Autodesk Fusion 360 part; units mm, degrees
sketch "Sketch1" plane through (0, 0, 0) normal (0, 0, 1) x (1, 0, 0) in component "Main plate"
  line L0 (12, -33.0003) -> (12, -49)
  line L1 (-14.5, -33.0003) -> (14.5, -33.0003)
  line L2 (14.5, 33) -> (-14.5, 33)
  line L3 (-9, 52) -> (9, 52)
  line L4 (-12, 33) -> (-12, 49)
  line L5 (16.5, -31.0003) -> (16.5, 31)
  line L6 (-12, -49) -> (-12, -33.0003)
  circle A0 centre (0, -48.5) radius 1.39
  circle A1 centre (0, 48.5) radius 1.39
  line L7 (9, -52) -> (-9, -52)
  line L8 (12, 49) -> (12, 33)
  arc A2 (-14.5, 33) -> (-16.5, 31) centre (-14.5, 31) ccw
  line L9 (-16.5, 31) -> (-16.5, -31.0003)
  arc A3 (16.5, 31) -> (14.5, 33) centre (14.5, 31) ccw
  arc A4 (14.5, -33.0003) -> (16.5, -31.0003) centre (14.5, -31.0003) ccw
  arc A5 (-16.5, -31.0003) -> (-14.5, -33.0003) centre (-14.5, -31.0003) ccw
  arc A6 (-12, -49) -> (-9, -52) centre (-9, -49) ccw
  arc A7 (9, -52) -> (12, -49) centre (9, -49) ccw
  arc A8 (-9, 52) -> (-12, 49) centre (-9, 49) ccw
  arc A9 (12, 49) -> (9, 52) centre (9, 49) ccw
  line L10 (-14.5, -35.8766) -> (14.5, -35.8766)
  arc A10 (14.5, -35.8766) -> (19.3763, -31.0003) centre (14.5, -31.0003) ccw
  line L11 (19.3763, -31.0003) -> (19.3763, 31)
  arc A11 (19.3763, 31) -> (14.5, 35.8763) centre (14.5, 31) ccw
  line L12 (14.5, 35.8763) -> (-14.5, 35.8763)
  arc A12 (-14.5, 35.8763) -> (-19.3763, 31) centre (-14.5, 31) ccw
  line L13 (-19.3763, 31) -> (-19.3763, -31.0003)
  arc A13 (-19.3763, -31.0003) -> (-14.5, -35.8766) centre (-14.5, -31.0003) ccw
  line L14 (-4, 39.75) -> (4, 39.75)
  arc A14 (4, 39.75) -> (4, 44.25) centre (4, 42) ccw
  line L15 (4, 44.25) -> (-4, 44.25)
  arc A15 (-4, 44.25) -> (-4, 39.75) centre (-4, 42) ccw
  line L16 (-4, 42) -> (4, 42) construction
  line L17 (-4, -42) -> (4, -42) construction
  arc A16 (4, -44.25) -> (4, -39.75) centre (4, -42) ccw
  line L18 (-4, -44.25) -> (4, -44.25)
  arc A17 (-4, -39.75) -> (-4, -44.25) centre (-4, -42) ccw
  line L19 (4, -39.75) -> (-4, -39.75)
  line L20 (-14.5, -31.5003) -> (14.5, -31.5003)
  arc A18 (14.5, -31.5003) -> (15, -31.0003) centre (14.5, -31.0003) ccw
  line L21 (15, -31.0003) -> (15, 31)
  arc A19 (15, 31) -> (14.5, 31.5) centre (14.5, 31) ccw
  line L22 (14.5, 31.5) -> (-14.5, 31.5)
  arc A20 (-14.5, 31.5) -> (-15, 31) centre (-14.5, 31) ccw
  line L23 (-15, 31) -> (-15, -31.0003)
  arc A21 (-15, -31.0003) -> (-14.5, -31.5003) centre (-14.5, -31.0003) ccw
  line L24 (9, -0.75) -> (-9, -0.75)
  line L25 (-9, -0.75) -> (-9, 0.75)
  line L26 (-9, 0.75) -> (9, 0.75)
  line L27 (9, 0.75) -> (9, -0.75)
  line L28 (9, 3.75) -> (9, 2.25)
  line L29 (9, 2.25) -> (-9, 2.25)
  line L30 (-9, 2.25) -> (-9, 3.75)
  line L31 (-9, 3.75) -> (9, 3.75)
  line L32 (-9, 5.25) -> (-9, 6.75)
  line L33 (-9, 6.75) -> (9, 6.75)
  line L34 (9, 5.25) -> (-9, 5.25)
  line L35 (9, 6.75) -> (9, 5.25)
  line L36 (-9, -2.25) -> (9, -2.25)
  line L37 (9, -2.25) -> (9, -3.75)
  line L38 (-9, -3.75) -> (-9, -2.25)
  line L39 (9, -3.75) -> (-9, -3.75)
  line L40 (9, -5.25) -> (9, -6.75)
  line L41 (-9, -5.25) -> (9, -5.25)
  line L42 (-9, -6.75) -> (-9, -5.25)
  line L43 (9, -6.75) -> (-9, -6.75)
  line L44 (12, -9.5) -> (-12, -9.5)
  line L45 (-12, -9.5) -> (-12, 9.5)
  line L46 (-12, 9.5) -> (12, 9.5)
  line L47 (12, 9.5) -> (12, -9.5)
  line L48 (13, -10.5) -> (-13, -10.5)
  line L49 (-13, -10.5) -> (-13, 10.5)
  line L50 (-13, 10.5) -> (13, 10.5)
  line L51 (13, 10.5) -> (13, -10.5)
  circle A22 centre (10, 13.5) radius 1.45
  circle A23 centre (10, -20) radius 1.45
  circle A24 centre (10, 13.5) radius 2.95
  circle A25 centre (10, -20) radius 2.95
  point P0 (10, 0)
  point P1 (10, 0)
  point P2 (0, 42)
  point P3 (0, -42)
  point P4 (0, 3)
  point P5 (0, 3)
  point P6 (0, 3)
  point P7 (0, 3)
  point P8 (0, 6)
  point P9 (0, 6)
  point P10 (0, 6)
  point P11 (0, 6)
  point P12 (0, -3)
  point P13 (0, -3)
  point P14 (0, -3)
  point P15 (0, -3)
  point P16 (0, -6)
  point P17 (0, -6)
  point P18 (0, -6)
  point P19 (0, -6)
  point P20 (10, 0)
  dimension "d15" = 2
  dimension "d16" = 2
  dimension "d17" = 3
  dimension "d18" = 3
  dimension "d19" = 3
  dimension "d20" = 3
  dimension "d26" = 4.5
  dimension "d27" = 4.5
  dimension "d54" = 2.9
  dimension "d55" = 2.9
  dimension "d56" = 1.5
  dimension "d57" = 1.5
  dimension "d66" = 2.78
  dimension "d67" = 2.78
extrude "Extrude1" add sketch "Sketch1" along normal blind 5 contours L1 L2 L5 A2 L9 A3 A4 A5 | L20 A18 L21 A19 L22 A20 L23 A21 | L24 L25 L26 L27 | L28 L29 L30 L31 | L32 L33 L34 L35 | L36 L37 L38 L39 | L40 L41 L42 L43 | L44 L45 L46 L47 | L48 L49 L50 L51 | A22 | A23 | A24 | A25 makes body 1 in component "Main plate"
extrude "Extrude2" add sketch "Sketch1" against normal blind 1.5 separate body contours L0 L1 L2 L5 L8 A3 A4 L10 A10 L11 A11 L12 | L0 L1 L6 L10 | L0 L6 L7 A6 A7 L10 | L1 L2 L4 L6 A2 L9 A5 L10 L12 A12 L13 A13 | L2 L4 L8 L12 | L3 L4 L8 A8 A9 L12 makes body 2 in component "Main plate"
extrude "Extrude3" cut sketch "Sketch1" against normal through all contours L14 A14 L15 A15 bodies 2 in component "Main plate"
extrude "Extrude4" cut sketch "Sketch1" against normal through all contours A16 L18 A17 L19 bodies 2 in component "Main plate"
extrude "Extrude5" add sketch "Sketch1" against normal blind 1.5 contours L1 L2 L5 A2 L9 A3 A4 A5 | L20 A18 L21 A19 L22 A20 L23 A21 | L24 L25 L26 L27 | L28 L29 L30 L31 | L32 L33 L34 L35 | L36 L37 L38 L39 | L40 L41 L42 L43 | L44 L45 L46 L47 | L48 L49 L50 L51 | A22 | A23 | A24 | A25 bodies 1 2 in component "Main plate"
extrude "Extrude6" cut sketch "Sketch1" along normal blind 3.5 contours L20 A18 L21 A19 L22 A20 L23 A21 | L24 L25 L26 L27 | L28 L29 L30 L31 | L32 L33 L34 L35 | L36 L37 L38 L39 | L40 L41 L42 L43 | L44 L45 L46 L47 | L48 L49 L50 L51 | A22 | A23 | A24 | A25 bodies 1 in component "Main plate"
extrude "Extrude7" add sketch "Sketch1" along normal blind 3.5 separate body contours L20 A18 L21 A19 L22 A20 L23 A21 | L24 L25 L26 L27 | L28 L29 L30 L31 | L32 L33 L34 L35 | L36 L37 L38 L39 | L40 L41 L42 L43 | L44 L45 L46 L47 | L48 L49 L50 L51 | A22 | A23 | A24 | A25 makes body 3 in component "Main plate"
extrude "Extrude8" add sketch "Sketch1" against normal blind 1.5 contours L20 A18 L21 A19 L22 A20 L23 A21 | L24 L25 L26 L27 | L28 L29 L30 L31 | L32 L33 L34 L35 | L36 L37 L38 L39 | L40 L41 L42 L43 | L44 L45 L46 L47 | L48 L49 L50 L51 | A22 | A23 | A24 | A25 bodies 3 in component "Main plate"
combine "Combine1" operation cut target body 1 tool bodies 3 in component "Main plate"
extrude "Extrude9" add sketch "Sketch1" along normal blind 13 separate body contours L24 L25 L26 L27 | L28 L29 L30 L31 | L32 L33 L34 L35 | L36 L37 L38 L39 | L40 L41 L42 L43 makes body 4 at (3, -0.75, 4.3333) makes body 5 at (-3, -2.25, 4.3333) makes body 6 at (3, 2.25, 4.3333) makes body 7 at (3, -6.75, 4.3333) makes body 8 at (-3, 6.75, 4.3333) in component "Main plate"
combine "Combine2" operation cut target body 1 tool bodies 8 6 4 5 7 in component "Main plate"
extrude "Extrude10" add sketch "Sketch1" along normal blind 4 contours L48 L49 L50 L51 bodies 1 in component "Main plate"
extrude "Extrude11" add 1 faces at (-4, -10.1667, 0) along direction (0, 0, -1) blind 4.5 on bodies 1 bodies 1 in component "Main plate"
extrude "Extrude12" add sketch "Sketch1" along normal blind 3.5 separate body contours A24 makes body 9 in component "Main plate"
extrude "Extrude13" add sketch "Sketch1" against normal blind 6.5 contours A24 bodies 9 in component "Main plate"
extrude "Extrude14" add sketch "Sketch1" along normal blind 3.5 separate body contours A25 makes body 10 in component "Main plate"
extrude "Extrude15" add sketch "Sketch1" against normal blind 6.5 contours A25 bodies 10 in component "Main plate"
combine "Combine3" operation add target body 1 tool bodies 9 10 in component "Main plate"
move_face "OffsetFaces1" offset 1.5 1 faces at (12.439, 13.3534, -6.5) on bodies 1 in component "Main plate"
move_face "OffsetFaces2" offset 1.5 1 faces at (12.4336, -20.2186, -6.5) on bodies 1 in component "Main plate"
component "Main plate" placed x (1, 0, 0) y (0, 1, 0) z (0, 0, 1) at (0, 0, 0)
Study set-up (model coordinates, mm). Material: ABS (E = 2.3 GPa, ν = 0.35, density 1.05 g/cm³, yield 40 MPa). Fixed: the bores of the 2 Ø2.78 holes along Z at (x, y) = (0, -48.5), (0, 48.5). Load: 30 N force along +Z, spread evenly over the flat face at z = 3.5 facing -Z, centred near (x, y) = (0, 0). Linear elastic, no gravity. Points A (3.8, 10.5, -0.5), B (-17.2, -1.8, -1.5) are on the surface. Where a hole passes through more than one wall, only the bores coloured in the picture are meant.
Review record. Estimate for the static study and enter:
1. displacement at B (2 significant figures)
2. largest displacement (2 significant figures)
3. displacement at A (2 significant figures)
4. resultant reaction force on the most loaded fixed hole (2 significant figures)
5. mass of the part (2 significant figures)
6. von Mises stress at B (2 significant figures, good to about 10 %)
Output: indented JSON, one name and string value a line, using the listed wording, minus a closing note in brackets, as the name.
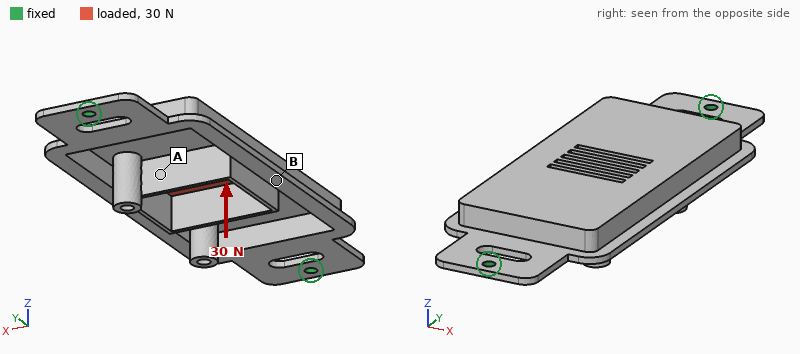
{
  "displacement at B": "1.1 mm",
  "largest displacement": "1.3 mm",
  "displacement at A": "1.2 mm",
  "resultant reaction force on the most loaded fixed hole": "41 N",
  "mass of the part": "7.9 g",
  "von Mises stress at B": "4.4 MPa"
}
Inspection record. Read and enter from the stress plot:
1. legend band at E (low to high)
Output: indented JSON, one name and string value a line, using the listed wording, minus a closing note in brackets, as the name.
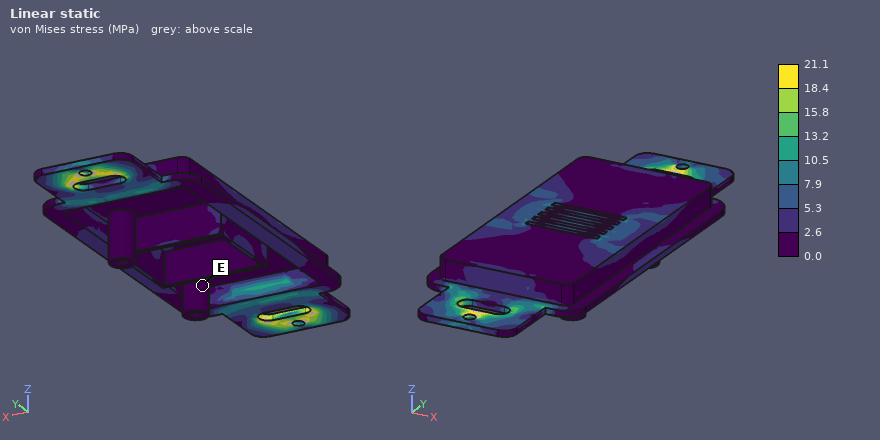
{
  "legend band at E": "0.0 to 2.6 MPa"
}
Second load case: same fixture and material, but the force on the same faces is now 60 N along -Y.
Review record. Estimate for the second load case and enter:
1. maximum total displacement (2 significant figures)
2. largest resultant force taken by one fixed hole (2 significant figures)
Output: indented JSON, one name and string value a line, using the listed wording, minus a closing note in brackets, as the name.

{
  "maximum total displacement": "0.18 mm",
  "largest resultant force taken by one fixed hole": "30 N"
}
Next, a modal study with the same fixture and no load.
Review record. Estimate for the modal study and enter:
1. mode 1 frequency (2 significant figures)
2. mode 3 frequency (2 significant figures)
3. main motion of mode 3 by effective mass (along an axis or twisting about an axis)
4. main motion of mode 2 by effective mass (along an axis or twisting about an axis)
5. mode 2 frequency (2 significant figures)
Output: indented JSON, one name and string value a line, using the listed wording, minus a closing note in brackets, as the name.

{
  "mode 1 frequency": "250 Hz",
  "mode 3 frequency": "670 Hz",
  "main motion of mode 3 by effective mass": "twisting about X",
  "main motion of mode 2 by effective mass": "along Z",
  "mode 2 frequency": "340 Hz"
}
